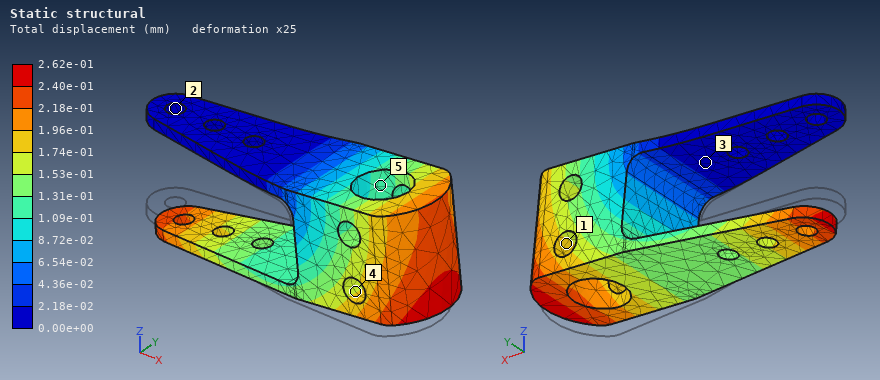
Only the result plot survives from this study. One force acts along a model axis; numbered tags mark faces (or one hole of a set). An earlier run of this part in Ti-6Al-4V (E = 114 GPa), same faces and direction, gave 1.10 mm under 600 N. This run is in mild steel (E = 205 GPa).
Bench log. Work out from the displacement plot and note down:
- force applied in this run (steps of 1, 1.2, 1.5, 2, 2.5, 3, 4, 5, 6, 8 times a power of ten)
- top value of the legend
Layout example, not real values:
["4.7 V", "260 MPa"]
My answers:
["250 N", "2.62e-01 mm"]
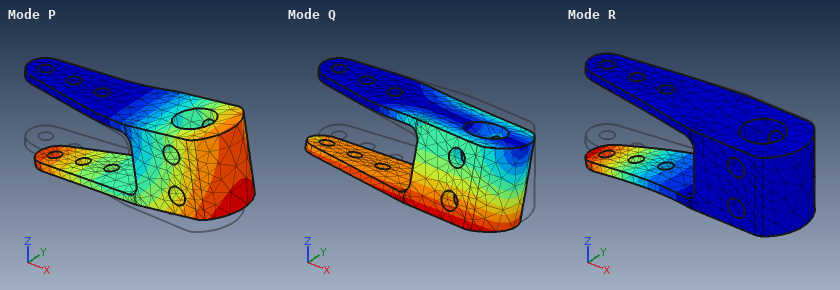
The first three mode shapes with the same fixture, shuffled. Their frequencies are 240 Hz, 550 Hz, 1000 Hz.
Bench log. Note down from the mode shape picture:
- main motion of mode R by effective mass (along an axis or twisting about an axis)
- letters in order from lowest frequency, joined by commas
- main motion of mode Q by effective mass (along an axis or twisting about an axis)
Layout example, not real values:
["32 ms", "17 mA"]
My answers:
["along Z", "P, Q, R", "along Y"]
